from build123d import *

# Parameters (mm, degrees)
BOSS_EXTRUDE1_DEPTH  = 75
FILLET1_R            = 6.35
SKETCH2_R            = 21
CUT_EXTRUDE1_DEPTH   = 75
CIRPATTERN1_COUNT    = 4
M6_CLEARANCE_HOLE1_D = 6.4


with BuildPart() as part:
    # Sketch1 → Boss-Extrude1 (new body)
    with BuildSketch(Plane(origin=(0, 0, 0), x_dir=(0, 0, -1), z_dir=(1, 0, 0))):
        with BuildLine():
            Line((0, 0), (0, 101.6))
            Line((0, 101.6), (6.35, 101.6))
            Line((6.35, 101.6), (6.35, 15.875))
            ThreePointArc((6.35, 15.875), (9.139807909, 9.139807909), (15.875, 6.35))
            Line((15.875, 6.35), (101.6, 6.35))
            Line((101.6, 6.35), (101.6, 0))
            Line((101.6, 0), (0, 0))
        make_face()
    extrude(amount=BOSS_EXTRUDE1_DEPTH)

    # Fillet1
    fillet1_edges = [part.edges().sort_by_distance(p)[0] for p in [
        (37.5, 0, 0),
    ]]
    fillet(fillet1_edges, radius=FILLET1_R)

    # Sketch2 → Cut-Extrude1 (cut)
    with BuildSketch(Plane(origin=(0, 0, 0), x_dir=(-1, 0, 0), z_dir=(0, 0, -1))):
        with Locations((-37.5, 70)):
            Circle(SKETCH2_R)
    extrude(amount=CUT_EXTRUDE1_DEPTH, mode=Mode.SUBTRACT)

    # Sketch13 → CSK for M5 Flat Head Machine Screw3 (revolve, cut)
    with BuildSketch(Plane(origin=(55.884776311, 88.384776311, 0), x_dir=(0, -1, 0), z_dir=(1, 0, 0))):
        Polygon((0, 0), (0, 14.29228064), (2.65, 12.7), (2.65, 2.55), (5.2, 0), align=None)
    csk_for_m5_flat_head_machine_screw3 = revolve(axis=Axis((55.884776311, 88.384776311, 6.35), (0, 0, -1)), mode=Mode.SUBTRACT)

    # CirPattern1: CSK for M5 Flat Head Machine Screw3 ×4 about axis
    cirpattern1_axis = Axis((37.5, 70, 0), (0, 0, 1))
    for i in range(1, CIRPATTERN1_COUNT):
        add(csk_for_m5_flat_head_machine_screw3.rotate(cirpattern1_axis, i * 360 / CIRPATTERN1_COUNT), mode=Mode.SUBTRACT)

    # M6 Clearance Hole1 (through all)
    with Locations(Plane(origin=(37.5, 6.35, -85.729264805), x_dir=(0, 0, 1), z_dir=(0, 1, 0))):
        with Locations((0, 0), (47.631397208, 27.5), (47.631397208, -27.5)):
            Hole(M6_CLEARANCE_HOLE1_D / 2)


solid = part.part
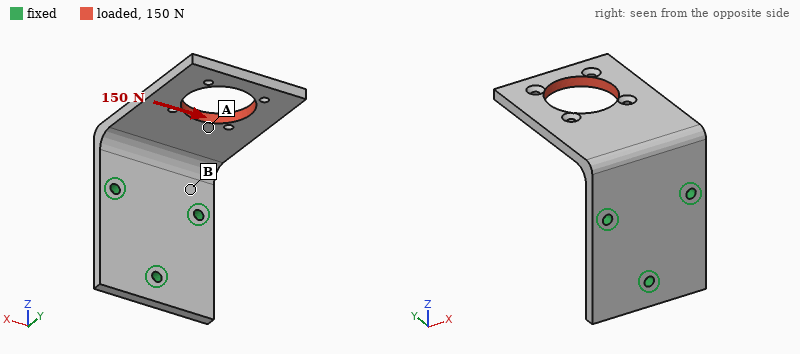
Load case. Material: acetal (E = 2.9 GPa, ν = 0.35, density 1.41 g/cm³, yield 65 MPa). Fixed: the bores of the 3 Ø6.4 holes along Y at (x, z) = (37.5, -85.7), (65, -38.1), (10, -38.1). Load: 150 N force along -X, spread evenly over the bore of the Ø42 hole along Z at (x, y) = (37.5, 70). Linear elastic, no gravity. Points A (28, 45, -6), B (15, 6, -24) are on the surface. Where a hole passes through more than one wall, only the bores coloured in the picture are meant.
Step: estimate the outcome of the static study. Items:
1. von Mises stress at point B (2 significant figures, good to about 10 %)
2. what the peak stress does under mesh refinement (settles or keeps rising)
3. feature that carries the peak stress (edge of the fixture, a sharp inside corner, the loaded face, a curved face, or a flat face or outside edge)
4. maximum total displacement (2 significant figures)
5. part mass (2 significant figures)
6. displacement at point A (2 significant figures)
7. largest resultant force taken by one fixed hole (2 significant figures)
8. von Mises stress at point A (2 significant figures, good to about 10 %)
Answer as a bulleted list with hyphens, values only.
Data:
- 7.2 MPa
- keeps rising
- edge of the fixture
- 1.7 mm
- 120 g
- 0.67 mm
- 210 N
- 2.0 MPa
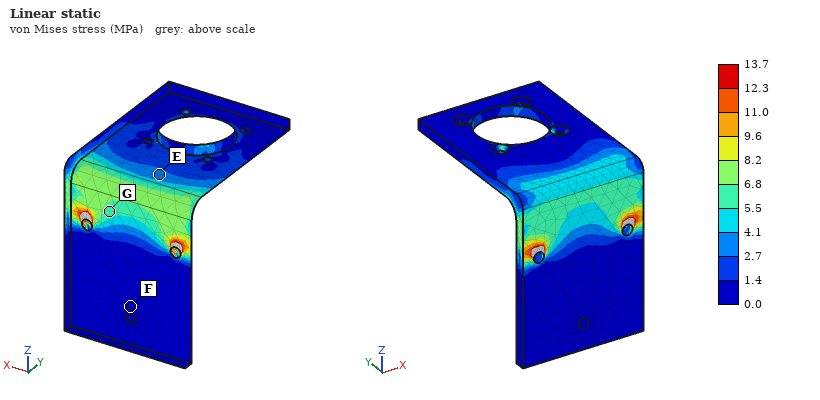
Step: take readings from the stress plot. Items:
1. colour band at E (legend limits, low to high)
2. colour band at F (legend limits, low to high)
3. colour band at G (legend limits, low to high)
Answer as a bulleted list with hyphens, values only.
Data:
- 2.7 to 4.1 MPa
- 0.0 to 1.4 MPa
- 5.5 to 6.8 MPa
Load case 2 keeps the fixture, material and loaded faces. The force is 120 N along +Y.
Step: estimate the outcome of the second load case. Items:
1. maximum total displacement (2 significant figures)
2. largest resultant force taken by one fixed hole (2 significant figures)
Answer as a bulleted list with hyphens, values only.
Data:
- 1.6 mm
- 70 N
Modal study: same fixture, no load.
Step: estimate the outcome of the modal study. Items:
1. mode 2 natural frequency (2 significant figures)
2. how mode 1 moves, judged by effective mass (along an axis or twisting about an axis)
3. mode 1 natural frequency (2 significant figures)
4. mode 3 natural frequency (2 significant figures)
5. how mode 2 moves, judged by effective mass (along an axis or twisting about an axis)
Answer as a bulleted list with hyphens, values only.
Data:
- 290 Hz
- along Z
- 120 Hz
- 420 Hz
- along X
